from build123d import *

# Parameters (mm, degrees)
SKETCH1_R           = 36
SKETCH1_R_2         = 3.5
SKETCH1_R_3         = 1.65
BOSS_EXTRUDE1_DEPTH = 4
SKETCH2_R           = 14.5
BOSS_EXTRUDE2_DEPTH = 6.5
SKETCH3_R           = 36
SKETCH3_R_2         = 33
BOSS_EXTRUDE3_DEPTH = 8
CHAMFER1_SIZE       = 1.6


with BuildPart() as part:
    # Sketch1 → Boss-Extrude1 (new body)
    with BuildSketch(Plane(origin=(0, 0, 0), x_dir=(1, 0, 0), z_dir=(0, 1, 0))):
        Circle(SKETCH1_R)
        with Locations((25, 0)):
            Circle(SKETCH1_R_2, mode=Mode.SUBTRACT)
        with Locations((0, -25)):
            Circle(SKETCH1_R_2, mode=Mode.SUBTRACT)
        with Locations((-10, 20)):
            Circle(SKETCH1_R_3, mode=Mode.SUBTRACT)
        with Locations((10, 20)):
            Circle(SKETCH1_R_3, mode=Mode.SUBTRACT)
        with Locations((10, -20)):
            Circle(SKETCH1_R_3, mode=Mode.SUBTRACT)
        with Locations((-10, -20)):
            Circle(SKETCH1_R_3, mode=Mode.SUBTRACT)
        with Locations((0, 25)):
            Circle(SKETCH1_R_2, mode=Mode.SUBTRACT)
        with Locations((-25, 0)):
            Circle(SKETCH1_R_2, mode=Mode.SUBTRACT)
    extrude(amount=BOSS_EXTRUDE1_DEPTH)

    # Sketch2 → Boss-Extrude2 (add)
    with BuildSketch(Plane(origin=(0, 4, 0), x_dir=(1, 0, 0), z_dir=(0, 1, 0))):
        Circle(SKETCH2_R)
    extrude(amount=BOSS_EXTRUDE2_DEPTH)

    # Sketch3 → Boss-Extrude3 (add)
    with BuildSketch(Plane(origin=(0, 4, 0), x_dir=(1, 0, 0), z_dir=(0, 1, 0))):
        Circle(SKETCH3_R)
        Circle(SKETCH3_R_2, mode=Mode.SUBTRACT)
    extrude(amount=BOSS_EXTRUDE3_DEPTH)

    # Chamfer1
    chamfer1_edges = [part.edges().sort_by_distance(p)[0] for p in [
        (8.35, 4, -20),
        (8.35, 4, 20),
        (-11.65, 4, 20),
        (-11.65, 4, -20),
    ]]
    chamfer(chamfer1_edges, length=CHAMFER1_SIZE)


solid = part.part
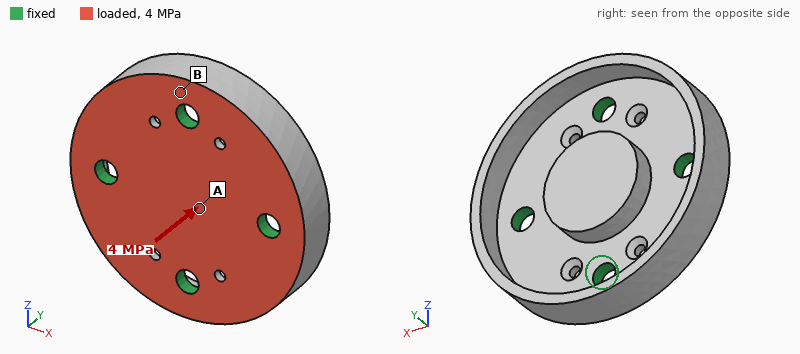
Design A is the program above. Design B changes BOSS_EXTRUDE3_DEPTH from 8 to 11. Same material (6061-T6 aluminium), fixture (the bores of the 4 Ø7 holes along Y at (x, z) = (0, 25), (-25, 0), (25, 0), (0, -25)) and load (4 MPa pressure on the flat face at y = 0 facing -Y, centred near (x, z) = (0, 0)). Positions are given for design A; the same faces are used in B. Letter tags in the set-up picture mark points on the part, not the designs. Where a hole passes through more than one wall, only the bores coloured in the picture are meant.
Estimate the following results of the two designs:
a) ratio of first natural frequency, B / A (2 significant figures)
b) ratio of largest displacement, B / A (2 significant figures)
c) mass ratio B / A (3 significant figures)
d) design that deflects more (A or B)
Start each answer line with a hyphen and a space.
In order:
- 0.86
- 0.82
- 1.08
- A
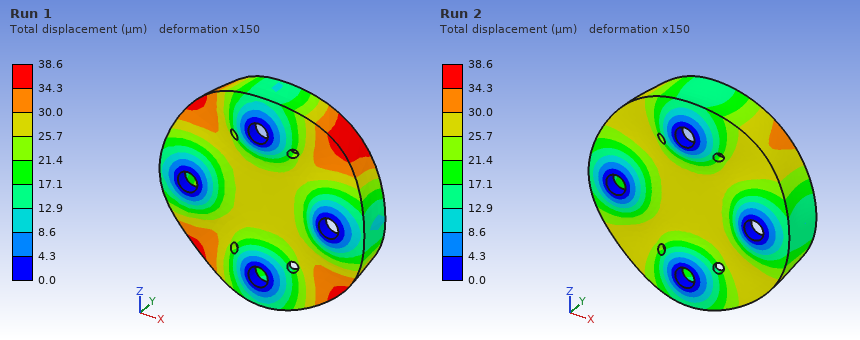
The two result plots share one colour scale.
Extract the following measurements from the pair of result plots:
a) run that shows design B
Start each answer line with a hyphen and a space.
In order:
- Run 2
